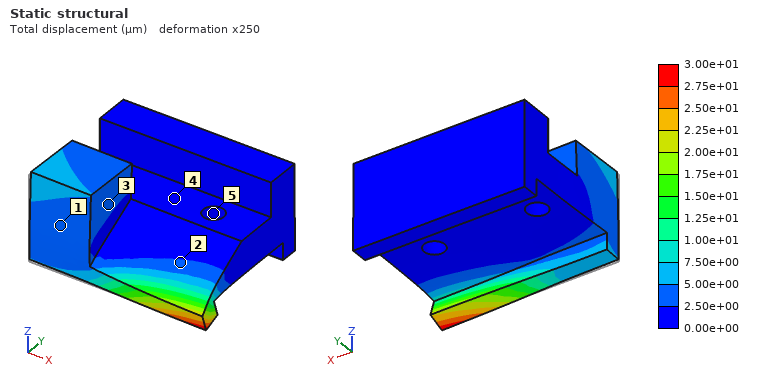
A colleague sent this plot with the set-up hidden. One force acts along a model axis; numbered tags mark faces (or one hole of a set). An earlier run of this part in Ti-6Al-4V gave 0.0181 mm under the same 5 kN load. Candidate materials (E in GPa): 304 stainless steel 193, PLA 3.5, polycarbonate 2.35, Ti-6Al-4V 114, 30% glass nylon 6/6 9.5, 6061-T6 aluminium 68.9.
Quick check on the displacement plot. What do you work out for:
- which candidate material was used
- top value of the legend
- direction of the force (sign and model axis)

6061-T6 aluminium
3.00e+01 µm
+Y
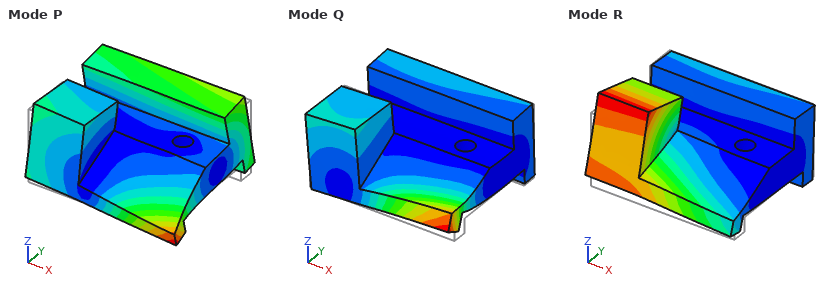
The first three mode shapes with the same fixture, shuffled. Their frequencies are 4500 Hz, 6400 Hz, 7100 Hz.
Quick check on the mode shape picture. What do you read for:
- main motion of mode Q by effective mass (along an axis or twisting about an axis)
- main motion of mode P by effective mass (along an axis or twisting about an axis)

along Z
along Z
